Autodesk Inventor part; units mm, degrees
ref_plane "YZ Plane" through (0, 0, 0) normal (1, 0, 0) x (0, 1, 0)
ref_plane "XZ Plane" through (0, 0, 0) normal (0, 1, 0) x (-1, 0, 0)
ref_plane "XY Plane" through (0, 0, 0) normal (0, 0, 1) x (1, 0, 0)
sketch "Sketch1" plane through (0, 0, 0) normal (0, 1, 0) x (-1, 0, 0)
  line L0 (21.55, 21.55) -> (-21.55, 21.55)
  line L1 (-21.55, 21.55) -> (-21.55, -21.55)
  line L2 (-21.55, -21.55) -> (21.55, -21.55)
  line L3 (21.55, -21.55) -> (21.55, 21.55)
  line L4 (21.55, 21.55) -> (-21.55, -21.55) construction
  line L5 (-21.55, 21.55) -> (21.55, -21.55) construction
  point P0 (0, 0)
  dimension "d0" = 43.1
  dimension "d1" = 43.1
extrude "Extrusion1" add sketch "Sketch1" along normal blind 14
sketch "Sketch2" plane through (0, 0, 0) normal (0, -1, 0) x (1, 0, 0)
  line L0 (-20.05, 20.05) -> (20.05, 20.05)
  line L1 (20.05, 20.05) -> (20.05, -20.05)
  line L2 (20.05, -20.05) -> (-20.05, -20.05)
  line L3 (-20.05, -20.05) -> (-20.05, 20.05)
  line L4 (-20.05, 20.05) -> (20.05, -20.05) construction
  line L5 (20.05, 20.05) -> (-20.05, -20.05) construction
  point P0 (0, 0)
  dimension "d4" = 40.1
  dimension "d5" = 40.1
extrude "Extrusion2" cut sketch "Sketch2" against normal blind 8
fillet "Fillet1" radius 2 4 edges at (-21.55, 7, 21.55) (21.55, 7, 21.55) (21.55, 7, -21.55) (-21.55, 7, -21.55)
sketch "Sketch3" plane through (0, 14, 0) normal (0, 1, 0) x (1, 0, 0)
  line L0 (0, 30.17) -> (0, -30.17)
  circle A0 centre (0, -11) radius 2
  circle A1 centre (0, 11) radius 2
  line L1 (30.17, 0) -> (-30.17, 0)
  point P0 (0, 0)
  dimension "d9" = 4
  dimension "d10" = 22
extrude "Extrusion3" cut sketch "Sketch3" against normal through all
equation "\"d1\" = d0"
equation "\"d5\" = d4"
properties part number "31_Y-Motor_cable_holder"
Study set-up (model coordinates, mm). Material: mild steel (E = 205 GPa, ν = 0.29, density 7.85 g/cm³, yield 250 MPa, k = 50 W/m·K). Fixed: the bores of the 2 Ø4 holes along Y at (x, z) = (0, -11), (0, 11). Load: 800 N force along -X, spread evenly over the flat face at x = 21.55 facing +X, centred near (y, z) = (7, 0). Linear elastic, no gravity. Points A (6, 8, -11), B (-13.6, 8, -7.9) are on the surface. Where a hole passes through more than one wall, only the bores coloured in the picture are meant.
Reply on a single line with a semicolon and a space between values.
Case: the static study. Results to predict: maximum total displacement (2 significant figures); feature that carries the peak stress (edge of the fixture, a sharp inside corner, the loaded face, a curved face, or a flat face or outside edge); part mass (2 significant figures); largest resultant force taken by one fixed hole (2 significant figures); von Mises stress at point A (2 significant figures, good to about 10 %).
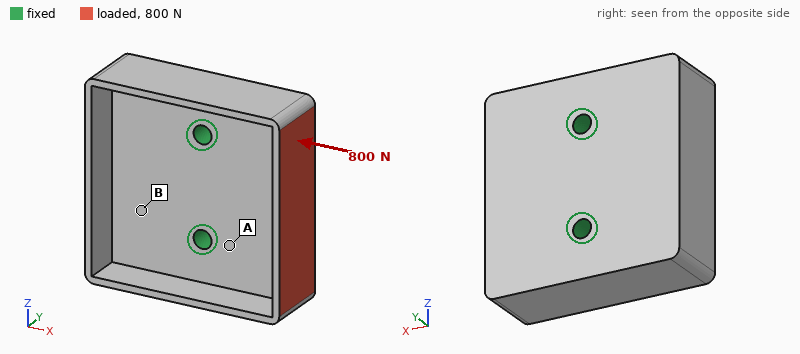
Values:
20 µm; the loaded face; 100 g; 410 N; 14 MPa
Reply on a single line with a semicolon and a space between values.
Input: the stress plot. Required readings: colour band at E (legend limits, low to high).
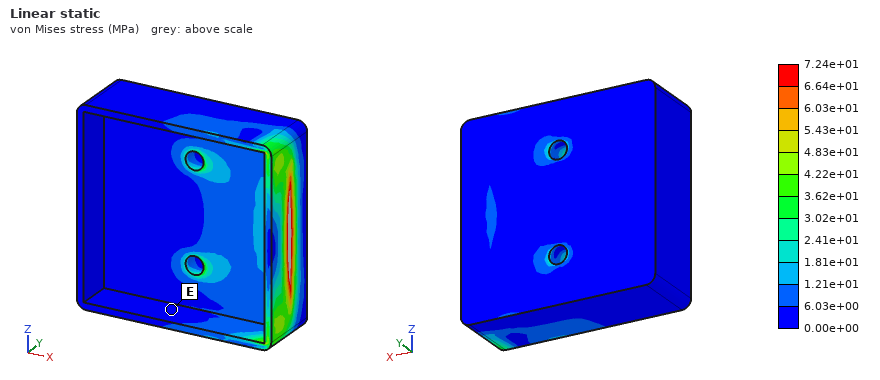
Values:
0.00e+00 to 6.03e+00 MPa
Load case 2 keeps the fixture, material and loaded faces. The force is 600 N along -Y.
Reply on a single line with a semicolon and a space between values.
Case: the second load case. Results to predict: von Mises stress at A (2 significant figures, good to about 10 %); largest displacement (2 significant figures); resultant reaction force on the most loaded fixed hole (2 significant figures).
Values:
31 MPa; 17 µm; 310 N
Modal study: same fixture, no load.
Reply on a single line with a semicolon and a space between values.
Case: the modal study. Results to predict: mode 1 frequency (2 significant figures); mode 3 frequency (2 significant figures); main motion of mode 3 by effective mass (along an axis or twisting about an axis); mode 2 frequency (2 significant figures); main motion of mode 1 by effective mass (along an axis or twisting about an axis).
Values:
7200 Hz; 11 kHz; along Y; 10 kHz; twisting about Z
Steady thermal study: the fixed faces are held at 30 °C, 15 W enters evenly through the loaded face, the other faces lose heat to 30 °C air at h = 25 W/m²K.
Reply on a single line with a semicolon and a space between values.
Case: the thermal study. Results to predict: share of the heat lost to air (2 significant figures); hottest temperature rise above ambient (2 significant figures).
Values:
9.4 %; 37 K
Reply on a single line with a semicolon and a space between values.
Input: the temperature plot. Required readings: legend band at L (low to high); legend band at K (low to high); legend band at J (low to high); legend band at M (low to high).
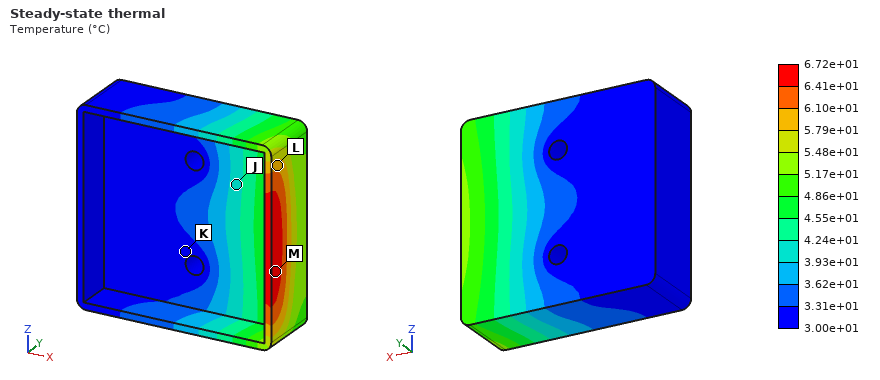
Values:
5.79e+01 to 6.10e+01 °C; 3.00e+01 to 3.31e+01 °C; 3.93e+01 to 4.24e+01 °C; 6.41e+01 to 6.72e+01 °C
